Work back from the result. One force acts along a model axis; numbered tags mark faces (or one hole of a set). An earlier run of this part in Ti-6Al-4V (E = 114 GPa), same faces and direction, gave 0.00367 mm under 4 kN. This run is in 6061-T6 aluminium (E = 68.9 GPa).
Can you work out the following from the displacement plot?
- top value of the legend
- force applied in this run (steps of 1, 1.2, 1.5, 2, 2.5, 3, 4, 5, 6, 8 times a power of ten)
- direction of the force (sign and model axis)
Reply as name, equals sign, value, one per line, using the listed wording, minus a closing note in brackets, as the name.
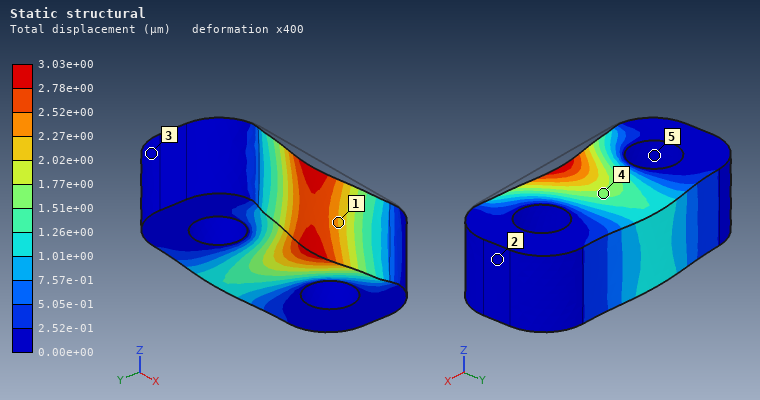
top value of the legend = 3.03e+00 µm
force applied in this run = 2 kN
direction of the force = +Y
